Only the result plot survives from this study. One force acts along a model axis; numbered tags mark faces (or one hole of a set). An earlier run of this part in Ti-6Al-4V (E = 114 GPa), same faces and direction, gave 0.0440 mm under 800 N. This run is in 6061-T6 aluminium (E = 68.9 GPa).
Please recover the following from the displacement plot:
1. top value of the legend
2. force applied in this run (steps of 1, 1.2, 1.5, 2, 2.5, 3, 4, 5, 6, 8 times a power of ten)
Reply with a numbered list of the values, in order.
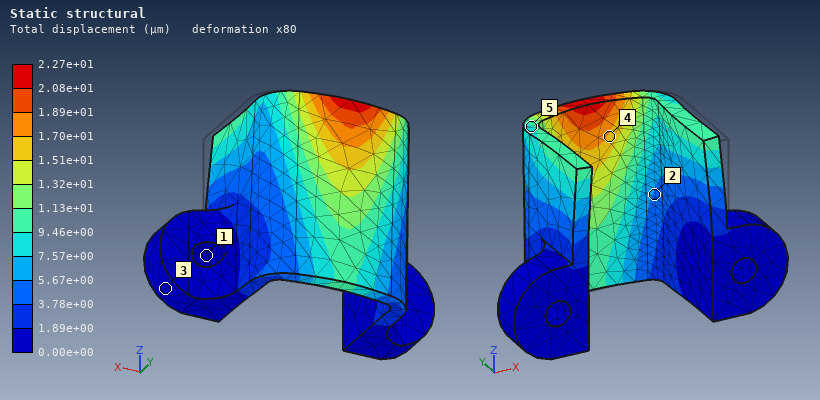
1. 2.27e+01 µm
2. 250 N
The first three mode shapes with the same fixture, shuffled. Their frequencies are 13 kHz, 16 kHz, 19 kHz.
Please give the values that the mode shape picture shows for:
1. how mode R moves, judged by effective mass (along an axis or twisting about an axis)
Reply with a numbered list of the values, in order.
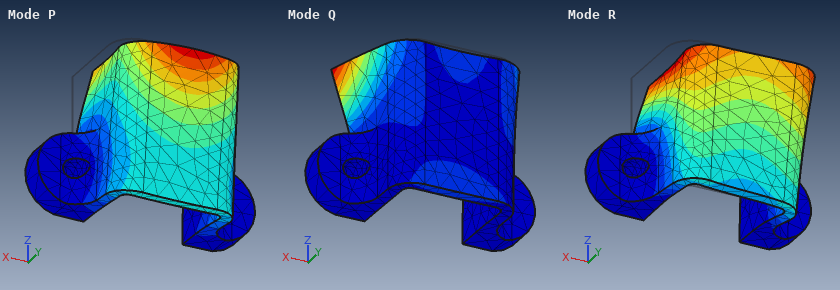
1. along X
